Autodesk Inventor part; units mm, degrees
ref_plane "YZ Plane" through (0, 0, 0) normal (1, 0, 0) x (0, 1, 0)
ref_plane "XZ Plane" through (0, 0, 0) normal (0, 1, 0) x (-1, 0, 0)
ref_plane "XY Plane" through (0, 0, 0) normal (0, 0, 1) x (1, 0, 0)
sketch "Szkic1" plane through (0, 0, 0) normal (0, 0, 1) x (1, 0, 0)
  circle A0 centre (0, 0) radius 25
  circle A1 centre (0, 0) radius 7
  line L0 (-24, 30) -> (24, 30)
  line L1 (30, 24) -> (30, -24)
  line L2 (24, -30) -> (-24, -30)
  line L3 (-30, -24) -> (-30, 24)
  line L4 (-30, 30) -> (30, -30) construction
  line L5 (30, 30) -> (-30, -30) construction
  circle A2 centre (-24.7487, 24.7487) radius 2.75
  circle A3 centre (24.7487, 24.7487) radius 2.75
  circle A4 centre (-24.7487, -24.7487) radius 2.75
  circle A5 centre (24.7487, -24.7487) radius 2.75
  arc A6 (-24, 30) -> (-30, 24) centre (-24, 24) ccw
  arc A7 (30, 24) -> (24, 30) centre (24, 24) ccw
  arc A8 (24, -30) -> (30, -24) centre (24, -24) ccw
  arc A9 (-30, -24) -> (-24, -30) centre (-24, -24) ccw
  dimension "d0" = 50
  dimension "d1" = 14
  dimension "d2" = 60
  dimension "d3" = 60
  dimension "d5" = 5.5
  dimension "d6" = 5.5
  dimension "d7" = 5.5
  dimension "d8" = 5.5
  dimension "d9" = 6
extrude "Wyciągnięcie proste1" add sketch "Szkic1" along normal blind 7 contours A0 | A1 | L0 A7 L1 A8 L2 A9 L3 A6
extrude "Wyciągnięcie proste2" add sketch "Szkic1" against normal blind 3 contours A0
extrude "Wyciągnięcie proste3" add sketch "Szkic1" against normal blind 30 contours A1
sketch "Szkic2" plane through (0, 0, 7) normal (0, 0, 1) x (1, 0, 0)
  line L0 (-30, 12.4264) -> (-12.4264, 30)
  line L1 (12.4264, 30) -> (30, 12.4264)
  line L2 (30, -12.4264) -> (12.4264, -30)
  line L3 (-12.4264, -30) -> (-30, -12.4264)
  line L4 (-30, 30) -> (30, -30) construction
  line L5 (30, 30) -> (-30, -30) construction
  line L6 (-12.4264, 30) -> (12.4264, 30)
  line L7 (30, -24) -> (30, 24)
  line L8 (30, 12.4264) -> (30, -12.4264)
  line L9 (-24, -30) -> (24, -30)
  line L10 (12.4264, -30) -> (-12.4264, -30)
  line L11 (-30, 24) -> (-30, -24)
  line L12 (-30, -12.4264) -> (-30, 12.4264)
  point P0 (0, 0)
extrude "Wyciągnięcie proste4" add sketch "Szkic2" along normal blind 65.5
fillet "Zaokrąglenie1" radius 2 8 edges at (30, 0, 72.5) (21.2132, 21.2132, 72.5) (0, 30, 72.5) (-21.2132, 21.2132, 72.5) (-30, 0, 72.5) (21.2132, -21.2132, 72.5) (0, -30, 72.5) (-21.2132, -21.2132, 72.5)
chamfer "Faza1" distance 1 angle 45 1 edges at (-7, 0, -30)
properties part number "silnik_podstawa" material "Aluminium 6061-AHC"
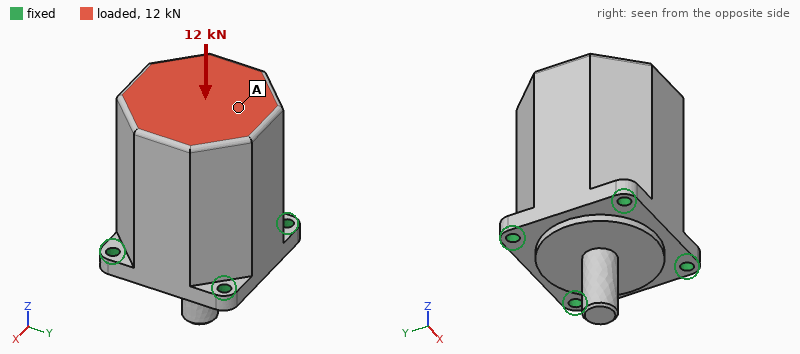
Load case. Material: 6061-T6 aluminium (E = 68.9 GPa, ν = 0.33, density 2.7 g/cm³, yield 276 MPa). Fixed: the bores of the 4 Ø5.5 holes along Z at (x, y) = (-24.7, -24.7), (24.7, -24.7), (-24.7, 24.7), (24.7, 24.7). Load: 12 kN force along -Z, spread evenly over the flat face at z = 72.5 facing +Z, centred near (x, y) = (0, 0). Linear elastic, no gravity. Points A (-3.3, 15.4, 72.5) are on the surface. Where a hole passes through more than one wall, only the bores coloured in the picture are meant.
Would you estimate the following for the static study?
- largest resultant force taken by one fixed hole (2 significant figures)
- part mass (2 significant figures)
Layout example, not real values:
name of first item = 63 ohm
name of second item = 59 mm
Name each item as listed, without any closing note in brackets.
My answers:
largest resultant force taken by one fixed hole = 3.2 kN
part mass = 620 g
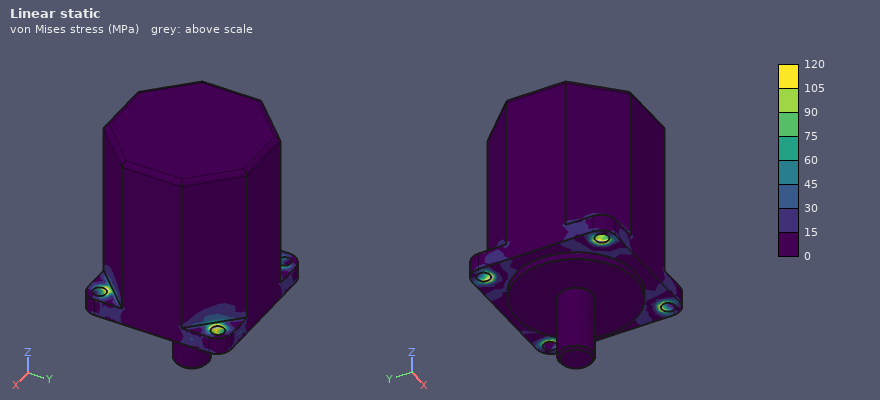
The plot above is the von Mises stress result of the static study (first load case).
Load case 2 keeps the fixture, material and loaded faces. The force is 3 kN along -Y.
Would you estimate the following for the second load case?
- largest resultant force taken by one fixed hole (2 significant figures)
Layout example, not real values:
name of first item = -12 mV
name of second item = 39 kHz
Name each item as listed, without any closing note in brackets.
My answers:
largest resultant force taken by one fixed hole = 2.5 kN
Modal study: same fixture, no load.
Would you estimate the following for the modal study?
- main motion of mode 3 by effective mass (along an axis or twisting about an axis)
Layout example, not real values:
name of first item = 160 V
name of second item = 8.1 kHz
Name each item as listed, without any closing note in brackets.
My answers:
main motion of mode 3 by effective mass = along Z
